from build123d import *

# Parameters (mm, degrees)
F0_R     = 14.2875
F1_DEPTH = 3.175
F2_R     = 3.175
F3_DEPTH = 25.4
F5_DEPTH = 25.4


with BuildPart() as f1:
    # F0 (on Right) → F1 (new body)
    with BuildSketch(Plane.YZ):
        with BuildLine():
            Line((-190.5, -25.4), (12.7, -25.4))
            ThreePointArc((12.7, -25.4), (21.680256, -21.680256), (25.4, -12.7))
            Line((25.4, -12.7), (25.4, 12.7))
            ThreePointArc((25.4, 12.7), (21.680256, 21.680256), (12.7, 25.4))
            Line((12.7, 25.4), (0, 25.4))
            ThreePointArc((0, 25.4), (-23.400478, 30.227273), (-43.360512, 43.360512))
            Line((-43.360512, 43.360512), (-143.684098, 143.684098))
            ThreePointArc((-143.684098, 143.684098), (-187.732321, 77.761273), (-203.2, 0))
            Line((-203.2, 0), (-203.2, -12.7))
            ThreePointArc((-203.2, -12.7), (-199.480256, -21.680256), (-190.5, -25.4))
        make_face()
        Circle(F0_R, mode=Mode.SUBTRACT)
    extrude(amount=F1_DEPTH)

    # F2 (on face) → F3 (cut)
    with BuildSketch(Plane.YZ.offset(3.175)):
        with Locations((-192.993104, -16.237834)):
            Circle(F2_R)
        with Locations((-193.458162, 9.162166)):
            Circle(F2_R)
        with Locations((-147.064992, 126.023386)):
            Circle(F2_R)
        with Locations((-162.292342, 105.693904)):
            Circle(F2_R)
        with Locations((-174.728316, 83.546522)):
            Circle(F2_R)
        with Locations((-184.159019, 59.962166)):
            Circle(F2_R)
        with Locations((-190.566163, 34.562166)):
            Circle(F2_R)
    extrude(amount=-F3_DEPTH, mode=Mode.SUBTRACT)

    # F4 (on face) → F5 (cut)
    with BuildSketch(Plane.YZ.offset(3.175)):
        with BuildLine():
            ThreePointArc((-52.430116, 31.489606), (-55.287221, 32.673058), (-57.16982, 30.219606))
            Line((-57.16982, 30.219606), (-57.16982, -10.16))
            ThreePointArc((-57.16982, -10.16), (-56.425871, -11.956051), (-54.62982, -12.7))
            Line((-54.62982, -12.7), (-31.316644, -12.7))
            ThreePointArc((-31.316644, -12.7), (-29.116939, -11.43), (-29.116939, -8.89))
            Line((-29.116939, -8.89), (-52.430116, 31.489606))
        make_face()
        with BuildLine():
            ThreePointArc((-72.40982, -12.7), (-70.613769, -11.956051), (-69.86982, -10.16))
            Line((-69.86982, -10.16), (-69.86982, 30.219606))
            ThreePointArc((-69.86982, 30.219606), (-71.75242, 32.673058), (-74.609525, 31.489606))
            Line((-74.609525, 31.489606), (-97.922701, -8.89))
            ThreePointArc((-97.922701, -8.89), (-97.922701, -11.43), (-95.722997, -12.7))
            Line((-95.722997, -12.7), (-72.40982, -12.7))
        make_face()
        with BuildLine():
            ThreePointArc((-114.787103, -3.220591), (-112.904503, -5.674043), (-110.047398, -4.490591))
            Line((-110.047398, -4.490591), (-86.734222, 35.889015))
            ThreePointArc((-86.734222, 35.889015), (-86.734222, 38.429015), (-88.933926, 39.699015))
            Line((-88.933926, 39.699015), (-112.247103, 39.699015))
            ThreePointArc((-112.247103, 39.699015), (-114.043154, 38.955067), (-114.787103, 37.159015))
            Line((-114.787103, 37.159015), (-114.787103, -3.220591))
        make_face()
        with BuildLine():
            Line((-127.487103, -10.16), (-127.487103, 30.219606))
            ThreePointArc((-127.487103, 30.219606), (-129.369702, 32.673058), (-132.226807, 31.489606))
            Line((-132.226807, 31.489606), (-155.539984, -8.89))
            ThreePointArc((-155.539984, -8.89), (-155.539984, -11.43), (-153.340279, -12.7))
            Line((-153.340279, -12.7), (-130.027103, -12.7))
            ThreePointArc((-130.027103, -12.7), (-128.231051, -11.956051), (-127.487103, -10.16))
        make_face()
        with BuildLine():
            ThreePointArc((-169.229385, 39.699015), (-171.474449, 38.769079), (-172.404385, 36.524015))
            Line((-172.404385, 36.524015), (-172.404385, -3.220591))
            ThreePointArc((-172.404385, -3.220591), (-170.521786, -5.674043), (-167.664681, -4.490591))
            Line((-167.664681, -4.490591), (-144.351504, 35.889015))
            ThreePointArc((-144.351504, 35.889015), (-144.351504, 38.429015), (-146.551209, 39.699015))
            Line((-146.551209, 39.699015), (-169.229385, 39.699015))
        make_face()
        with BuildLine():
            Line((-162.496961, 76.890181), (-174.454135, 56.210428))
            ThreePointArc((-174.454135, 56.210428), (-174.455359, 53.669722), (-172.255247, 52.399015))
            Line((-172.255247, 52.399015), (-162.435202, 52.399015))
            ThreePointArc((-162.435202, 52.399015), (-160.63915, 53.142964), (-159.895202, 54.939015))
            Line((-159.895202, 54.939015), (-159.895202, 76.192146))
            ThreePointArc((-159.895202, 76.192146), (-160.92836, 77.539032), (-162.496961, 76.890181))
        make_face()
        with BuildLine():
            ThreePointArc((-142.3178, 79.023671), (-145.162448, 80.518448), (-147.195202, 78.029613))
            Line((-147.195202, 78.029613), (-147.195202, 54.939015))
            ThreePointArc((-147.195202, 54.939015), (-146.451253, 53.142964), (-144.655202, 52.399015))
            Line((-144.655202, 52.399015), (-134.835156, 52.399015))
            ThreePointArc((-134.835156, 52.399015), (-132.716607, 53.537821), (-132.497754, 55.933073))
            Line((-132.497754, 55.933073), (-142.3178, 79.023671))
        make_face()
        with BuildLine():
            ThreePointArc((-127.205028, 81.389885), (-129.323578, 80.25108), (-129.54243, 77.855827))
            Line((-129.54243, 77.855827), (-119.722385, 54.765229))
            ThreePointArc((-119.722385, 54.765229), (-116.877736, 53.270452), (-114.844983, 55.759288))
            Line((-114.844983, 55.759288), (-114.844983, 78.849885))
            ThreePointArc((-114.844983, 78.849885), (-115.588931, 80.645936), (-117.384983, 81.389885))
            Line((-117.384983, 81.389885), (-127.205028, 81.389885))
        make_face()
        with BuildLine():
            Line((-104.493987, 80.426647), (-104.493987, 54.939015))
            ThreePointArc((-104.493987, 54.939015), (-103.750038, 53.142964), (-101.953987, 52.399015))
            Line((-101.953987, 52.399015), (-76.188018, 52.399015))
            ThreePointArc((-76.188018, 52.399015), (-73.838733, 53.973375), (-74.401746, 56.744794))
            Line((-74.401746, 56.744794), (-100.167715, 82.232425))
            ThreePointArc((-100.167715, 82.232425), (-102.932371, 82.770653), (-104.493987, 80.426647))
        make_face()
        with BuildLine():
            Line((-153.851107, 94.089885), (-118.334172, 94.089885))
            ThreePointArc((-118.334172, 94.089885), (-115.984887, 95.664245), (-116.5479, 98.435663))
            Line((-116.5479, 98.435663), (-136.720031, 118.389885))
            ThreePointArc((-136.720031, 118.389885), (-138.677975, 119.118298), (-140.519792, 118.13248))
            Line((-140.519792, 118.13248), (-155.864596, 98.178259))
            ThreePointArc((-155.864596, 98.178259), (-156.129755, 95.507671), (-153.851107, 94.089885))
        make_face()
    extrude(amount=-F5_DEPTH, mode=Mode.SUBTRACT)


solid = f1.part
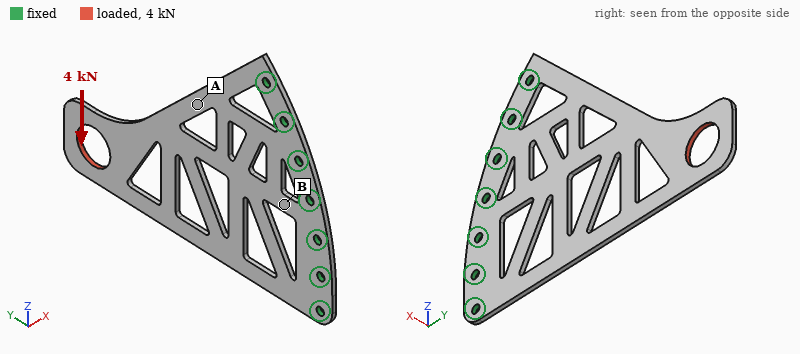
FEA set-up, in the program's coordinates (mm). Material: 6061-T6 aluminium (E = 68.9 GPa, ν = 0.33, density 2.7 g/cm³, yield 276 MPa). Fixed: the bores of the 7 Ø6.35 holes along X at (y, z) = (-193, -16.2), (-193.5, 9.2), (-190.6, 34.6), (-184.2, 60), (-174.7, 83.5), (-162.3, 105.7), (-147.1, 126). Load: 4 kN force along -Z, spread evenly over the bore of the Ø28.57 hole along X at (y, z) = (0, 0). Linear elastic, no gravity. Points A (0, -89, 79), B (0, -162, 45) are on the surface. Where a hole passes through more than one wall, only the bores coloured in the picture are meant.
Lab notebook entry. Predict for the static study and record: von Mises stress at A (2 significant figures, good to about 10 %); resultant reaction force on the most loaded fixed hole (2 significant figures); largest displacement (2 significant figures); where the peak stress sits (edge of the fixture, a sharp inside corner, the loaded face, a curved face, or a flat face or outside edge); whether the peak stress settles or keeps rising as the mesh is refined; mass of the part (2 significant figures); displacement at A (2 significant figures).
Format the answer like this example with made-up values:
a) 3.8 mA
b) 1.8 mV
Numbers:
a) 110 MPa
b) 4.2 kN
c) 0.79 mm
d) edge of the fixture
e) keeps rising
f) 140 g
g) 0.14 mm
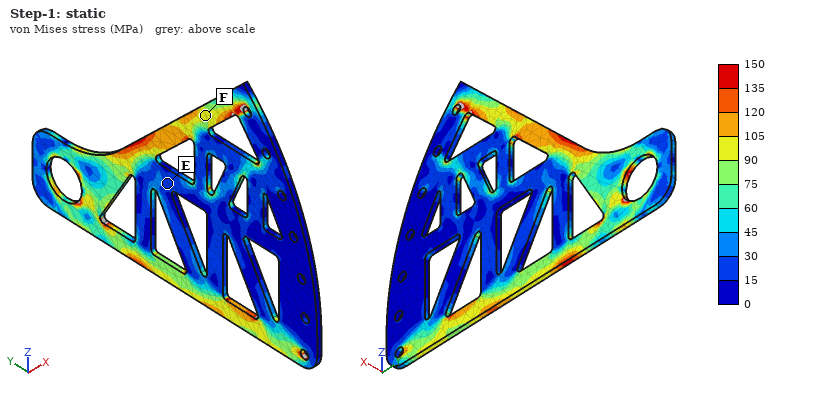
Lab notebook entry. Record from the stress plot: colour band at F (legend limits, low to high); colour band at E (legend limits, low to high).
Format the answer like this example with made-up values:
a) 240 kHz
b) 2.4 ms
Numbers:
a) 90 to 105 MPa
b) 15 to 30 MPa
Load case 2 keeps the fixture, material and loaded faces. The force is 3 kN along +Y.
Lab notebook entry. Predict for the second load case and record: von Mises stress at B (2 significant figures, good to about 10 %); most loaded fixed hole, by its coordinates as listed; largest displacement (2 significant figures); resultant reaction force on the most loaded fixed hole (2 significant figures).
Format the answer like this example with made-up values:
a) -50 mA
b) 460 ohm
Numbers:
a) 21 MPa
b) (-193, -16.2)
c) 0.18 mm
d) 1.9 kN
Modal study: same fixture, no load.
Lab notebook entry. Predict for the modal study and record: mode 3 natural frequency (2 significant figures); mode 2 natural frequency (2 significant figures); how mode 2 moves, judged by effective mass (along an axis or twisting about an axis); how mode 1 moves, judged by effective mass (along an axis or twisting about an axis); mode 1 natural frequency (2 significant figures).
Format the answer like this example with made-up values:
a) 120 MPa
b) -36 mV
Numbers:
a) 420 Hz
b) 340 Hz
c) along X
d) along X
e) 72 Hz
